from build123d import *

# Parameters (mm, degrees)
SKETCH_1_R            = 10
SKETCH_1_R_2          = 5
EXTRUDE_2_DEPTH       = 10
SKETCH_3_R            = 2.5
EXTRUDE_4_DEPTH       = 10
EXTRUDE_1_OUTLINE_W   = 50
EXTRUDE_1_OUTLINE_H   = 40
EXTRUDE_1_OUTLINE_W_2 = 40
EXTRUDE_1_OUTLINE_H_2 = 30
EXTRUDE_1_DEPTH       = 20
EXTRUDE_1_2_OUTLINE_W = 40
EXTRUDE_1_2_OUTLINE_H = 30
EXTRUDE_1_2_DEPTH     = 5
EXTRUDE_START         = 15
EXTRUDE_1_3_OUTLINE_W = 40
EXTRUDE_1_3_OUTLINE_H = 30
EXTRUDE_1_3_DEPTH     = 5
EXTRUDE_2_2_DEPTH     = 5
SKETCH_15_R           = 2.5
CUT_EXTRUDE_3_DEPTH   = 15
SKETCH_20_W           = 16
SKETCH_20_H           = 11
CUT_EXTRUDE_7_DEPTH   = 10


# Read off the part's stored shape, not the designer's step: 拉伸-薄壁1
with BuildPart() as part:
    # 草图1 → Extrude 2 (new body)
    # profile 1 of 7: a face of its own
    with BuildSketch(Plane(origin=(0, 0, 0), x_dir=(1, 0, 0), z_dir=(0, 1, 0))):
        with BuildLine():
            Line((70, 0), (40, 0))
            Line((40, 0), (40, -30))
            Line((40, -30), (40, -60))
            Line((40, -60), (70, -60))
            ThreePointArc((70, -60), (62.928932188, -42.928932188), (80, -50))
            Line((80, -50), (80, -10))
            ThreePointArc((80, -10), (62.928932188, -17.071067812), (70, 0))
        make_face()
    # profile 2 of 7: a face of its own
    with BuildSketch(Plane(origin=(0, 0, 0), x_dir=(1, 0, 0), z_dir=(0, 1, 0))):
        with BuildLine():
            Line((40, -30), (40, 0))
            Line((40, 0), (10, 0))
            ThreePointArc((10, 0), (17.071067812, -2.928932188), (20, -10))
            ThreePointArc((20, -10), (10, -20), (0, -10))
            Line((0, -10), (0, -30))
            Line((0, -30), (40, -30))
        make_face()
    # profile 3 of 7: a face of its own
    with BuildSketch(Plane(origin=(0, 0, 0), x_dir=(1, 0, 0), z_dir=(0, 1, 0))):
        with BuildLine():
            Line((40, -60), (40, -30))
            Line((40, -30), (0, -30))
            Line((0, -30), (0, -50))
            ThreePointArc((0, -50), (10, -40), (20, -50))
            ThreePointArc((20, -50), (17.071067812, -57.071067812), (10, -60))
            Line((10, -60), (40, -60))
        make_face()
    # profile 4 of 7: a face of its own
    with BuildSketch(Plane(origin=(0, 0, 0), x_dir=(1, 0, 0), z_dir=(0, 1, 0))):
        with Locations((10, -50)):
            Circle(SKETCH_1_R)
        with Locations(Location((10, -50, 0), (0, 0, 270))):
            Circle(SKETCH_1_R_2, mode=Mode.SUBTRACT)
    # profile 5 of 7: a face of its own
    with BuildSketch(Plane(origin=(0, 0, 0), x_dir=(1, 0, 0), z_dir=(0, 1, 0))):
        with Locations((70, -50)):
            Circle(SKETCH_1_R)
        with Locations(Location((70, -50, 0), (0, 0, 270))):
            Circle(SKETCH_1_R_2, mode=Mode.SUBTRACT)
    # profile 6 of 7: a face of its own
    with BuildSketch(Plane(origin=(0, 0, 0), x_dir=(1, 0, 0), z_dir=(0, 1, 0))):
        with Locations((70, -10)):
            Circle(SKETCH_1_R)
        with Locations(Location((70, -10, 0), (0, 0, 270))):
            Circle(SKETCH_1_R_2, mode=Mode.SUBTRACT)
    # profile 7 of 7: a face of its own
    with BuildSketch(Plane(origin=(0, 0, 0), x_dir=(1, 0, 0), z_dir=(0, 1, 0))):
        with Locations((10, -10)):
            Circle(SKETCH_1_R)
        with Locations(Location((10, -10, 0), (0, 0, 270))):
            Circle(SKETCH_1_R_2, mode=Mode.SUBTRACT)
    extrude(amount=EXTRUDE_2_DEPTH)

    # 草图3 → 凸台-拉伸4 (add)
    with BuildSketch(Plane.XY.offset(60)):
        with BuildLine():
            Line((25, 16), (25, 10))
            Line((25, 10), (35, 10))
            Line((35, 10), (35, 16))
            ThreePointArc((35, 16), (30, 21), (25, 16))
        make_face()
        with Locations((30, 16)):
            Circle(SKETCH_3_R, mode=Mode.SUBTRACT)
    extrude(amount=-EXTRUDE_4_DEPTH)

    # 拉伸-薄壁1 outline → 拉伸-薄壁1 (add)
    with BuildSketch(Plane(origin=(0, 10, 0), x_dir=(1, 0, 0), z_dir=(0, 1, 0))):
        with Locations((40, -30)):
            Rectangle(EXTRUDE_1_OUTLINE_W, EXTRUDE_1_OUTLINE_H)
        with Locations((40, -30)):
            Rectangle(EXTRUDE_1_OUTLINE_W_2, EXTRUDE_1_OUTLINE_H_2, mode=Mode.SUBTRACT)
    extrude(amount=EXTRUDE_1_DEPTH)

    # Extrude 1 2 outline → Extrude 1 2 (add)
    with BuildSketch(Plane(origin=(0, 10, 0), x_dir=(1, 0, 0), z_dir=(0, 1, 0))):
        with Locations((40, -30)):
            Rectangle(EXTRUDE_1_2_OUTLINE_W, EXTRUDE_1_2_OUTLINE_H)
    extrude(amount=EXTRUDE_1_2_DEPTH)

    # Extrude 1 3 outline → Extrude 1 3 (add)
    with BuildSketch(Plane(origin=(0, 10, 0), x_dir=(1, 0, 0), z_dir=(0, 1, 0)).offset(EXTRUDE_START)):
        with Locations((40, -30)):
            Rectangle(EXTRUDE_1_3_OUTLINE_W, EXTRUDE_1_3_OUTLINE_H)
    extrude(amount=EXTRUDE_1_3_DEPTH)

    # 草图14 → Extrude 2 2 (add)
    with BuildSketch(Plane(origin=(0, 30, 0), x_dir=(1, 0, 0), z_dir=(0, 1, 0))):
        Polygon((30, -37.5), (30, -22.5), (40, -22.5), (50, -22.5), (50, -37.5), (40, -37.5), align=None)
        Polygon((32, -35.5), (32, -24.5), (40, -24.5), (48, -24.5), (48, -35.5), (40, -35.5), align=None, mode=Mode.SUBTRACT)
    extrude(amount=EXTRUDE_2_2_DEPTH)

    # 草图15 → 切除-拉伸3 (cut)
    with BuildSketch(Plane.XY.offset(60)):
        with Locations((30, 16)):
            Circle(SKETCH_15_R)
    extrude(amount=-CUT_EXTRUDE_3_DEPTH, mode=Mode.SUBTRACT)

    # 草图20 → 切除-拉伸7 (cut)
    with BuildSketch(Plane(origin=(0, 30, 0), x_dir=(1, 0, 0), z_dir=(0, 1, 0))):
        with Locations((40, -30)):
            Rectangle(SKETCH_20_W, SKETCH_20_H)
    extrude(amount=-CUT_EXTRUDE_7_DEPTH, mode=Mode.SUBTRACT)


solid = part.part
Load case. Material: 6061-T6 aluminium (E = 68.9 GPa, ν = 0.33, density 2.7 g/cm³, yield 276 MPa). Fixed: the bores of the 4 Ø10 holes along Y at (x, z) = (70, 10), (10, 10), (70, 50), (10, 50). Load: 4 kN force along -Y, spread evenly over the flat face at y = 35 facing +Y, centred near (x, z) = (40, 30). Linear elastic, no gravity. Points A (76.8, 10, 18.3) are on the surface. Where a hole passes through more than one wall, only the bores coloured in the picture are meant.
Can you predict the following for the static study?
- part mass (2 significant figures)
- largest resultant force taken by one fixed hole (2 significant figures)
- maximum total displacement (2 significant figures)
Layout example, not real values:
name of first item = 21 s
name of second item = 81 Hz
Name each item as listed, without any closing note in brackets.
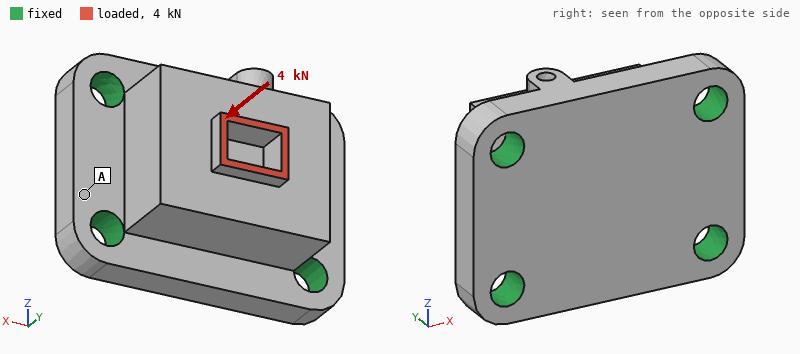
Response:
part mass = 200 g
largest resultant force taken by one fixed hole = 1.1 kN
maximum total displacement = 35 µm
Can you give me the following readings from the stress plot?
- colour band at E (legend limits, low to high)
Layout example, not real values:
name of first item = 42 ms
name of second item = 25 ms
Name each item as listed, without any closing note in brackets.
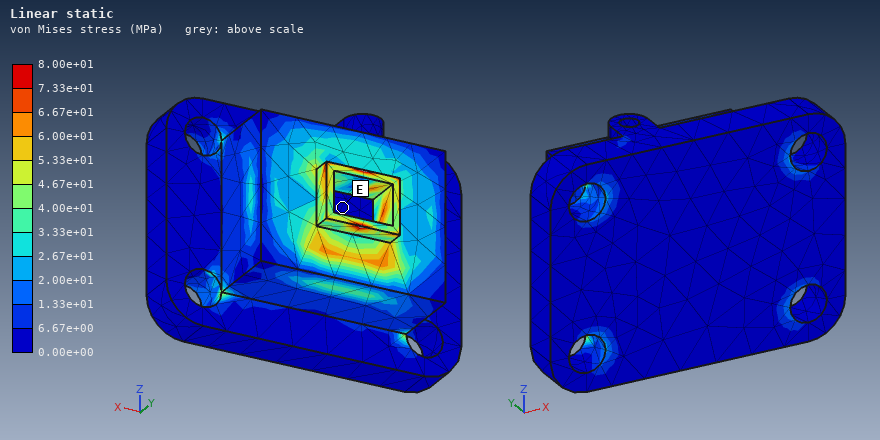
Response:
colour band at E = 0.00e+00 to 6.67e+00 MPa
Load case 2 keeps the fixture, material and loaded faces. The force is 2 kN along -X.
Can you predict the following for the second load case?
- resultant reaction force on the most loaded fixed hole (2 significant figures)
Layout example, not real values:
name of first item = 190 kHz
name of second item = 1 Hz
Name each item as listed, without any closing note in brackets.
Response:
resultant reaction force on the most loaded fixed hole = 780 N
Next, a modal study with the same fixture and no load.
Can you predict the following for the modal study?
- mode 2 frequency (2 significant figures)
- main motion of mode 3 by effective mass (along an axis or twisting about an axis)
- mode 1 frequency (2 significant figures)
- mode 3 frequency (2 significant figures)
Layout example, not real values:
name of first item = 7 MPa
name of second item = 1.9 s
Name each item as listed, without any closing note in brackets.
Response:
mode 2 frequency = 15 kHz
main motion of mode 3 by effective mass = along X
mode 1 frequency = 14 kHz
mode 3 frequency = 18 kHz
